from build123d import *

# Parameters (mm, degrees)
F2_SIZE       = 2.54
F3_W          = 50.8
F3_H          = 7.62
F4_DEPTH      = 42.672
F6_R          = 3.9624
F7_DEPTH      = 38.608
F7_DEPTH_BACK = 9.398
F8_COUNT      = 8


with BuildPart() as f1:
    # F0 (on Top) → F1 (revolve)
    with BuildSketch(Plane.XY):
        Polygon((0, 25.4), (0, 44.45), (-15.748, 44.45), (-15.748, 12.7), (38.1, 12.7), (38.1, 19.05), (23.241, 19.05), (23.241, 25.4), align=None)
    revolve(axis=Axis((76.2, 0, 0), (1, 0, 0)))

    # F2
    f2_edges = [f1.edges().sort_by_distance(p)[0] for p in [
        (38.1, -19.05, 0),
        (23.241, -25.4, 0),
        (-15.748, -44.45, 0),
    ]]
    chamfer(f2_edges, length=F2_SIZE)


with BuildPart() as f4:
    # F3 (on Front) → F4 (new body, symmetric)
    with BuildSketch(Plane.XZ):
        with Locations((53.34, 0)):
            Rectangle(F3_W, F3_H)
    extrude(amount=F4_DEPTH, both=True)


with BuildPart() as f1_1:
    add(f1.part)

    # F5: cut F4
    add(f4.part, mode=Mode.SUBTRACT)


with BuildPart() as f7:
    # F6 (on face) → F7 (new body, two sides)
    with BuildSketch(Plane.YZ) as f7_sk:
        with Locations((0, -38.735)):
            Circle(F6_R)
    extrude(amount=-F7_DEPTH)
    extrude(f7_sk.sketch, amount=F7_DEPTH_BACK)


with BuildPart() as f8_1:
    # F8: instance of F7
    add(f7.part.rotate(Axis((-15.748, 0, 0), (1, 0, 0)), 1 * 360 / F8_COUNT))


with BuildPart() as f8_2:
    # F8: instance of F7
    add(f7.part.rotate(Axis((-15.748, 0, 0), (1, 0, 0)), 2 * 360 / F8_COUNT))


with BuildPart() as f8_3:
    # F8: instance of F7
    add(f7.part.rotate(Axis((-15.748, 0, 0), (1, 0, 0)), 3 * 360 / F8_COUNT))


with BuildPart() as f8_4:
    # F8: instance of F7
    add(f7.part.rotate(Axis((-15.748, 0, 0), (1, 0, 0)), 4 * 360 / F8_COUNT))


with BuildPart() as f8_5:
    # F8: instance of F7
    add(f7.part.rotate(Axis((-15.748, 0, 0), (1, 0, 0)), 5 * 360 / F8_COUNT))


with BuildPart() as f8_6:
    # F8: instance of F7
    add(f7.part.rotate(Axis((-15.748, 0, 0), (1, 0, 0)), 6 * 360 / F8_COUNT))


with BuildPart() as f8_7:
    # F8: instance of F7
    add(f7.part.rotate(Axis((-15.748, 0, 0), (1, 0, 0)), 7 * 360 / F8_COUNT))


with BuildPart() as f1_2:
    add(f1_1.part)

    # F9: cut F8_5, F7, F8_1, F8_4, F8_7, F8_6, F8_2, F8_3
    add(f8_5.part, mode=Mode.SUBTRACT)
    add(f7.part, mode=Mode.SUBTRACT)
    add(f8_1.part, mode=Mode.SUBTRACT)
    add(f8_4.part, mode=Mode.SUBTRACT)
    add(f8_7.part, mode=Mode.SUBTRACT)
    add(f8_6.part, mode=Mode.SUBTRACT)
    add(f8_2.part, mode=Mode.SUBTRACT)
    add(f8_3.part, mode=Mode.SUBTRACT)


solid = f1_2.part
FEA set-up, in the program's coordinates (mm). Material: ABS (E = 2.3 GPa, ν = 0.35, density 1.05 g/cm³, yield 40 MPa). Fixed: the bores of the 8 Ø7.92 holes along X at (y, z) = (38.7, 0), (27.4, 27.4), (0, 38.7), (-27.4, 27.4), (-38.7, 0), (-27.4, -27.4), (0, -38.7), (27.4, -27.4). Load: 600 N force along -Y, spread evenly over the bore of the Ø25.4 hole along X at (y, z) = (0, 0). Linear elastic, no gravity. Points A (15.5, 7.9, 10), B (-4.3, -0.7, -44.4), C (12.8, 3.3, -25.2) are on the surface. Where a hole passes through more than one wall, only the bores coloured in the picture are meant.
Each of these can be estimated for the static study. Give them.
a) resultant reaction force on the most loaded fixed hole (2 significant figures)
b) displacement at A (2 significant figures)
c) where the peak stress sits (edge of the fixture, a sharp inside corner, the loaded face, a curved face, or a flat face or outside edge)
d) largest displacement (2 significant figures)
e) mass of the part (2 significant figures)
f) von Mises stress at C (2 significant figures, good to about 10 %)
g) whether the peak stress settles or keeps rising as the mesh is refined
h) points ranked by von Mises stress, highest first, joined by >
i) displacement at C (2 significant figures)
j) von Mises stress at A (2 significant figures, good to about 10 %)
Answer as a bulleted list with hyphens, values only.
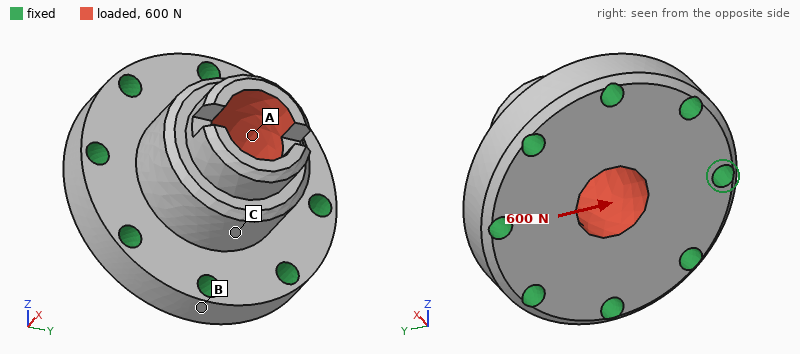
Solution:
- 150 N
- 14 µm
- edge of the fixture
- 37 µm
- 130 g
- 0.26 MPa
- keeps rising
- A > C > B
- 11 µm
- 0.70 MPa
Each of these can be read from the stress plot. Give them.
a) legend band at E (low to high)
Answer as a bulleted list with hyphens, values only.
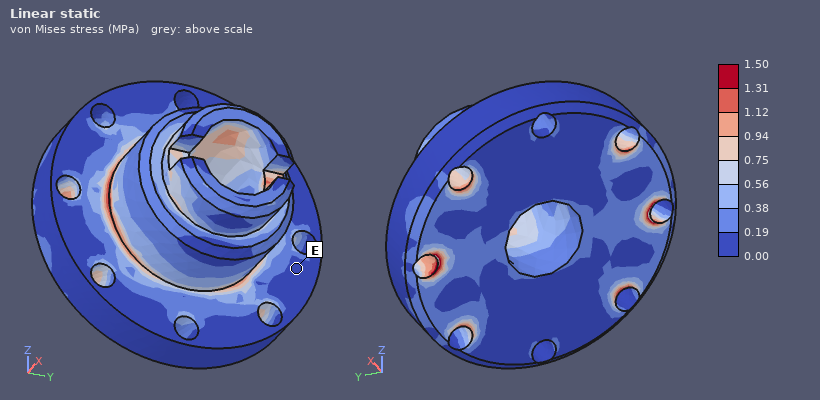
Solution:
- 0.00 to 0.19 MPa
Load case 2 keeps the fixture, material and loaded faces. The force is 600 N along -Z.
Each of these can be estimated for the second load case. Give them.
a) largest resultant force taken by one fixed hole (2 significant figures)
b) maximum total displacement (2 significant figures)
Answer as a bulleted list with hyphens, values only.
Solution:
- 150 N
- 33 µm
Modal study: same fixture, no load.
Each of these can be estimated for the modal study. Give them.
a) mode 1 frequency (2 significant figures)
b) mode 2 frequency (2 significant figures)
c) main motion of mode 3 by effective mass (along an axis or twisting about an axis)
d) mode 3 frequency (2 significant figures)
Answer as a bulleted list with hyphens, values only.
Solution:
- 3900 Hz
- 3900 Hz
- along X
- 4900 Hz
